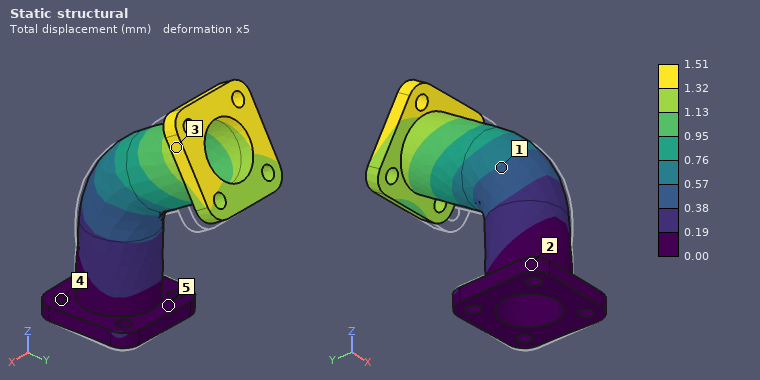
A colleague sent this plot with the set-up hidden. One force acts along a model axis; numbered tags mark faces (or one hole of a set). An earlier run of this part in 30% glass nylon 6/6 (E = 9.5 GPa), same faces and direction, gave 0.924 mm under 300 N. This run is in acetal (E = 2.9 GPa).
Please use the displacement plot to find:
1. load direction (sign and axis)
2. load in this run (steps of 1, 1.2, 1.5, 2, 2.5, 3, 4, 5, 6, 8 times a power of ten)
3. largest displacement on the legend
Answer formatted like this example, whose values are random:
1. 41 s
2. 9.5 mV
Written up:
1. -X
2. 150 N
3. 1.51 mm
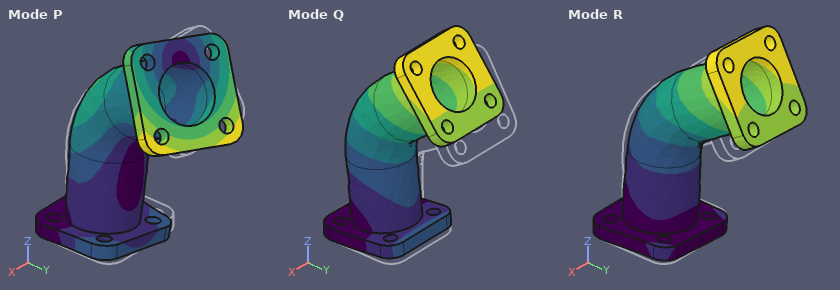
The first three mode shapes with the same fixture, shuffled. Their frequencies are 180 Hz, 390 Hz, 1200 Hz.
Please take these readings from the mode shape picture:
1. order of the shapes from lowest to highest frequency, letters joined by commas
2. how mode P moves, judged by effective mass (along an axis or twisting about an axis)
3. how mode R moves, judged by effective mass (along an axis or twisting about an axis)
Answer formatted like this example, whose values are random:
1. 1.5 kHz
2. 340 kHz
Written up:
1. Q, R, P
2. twisting about Z
3. along X
